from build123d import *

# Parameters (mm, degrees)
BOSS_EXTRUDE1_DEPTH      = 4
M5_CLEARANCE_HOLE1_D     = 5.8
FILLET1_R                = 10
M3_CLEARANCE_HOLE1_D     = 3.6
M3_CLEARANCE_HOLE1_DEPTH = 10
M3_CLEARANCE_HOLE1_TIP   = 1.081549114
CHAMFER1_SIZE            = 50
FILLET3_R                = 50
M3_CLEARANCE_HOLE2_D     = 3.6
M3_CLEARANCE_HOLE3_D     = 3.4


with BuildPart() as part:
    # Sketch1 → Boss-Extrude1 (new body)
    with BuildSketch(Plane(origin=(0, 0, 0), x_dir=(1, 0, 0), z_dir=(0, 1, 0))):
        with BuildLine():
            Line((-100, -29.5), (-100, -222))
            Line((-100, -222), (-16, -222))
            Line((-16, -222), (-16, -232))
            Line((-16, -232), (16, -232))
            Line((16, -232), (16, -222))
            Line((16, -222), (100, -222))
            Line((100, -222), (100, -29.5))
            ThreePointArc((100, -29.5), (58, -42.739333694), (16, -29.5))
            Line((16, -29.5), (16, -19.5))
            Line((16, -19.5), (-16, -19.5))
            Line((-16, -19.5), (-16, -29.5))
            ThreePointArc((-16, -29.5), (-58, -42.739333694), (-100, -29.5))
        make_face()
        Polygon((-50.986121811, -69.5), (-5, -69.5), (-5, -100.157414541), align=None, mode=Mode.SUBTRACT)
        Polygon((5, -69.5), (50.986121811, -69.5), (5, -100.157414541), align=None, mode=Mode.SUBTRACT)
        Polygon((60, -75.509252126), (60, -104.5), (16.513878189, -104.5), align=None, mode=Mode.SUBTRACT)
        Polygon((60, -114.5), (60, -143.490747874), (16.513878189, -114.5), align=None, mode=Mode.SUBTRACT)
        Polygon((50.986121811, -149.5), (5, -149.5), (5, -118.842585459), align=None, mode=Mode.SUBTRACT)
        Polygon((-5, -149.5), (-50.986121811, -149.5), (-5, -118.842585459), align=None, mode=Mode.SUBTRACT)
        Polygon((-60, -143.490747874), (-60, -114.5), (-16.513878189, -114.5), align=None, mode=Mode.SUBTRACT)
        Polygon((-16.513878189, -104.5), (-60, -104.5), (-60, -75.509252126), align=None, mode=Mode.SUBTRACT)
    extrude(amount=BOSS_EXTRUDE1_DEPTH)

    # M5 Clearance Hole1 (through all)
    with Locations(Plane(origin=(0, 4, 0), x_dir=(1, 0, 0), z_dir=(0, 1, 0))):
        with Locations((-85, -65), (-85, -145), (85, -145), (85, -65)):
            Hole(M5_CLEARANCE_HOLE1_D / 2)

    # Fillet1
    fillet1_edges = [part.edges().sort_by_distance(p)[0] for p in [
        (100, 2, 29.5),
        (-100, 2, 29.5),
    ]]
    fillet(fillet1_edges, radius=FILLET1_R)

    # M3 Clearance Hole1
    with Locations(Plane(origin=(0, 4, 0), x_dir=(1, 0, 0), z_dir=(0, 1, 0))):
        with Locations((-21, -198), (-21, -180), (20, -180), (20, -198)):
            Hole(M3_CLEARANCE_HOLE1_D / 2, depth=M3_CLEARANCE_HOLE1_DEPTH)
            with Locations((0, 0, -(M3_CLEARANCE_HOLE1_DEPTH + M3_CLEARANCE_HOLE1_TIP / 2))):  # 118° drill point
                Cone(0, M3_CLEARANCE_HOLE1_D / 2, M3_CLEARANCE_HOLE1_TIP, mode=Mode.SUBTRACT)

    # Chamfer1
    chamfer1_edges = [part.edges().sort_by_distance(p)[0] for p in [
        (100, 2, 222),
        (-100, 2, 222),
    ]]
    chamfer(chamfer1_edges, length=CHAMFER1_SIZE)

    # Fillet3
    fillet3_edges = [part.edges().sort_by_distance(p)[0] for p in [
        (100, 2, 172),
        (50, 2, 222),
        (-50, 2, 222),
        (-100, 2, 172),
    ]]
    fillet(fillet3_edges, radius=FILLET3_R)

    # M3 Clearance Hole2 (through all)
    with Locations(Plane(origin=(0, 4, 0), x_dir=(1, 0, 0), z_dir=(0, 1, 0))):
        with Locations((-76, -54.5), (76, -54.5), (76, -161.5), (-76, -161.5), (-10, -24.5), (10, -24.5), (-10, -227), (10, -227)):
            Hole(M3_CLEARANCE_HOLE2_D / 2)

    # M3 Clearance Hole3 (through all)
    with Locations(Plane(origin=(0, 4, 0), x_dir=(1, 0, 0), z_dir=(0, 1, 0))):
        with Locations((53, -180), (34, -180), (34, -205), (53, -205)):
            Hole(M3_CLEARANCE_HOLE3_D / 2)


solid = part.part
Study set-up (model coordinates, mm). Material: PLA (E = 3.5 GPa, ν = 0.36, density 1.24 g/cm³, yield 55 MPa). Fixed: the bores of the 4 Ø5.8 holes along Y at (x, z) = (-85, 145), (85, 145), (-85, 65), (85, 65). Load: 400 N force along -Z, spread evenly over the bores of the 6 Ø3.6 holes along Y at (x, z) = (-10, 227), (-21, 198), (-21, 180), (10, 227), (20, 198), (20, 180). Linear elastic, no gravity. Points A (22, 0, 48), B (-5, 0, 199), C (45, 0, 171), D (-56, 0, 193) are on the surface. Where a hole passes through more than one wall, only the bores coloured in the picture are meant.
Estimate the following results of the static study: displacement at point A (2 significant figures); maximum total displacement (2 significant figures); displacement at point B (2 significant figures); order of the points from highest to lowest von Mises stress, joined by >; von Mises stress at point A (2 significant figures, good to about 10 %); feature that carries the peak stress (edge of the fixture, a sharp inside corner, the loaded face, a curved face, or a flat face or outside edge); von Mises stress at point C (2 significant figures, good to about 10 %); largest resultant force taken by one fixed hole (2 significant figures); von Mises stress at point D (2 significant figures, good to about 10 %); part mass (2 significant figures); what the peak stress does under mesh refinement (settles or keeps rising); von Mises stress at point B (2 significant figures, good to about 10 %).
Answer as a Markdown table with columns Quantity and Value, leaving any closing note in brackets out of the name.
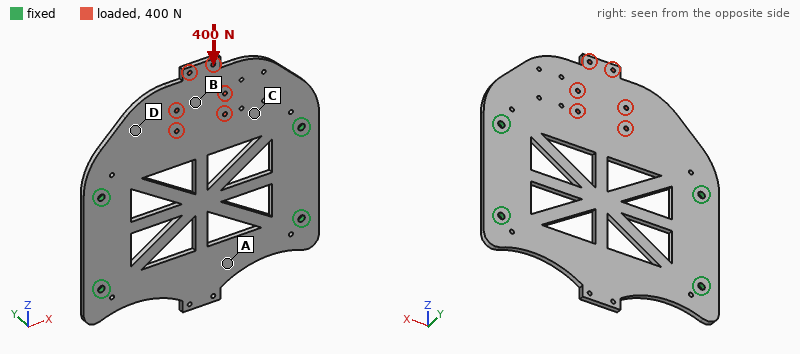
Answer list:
| Quantity | Value |
|---|---|
| displacement at point A | 15 µm |
| maximum total displacement | 61 µm |
| displacement at point B | 55 µm |
| order of the points from highest to lowest von Mises stress, joined by > | C > D > B > A |
| von Mises stress at point A | 0.24 MPa |
| feature that carries the peak stress | edge of the fixture |
| von Mises stress at point C | 1.3 MPa |
| largest resultant force taken by one fixed hole | 170 N |
| von Mises stress at point D | 0.91 MPa |
| part mass | 140 g |
| what the peak stress does under mesh refinement | keeps rising |
| von Mises stress at point B | 0.60 MPa |
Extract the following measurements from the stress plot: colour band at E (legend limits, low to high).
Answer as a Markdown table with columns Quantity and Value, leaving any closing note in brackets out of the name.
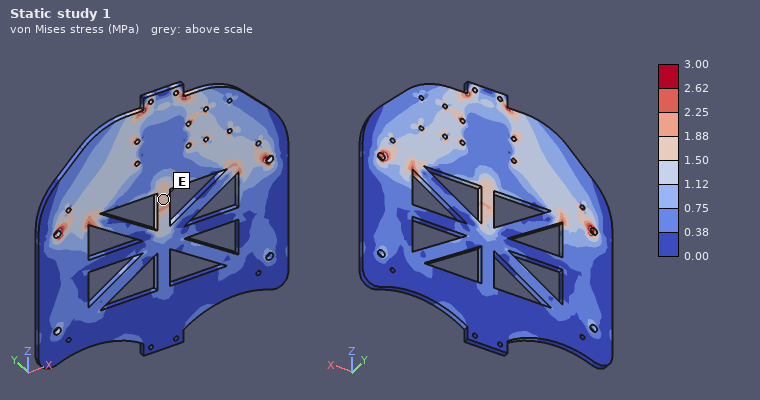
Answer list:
| Quantity | Value |
|---|---|
| colour band at E | 1.50 to 1.88 MPa |
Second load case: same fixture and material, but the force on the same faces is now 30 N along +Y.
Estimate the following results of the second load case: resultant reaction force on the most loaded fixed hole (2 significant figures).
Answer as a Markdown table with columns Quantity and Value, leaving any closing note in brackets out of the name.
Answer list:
| Quantity | Value |
|---|---|
| resultant reaction force on the most loaded fixed hole | 19 N |
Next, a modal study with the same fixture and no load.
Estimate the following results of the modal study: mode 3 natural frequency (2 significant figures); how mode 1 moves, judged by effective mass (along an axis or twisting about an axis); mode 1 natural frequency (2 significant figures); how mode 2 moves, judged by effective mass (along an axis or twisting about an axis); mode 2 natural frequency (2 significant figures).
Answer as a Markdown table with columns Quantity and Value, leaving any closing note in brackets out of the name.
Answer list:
| Quantity | Value |
|---|---|
| mode 3 natural frequency | 290 Hz |
| how mode 1 moves, judged by effective mass | along Y |
| mode 1 natural frequency | 120 Hz |
| how mode 2 moves, judged by effective mass | along Y |
| mode 2 natural frequency | 210 Hz |
